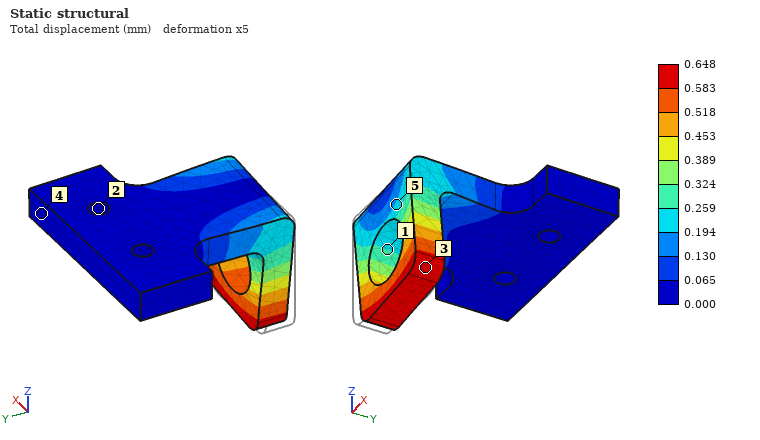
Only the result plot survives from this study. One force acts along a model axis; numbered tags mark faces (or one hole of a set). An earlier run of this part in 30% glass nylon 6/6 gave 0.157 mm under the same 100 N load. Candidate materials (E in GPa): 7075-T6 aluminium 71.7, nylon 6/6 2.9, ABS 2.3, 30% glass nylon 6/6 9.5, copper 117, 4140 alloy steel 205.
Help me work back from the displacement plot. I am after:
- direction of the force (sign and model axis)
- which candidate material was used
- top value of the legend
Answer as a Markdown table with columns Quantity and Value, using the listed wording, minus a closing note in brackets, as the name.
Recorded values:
| Quantity | Value |
|---|---|
| direction of the force | +X |
| which candidate material was used | ABS |
| top value of the legend | 0.648 mm |
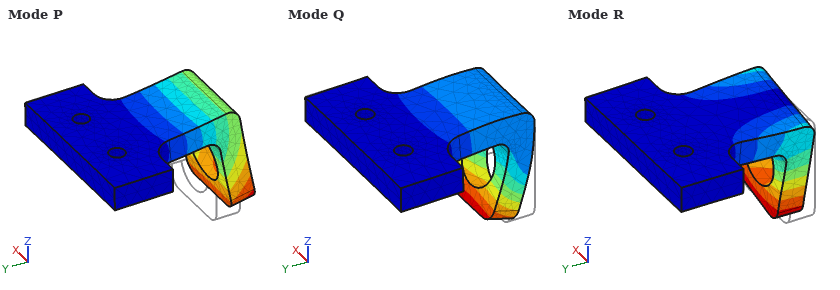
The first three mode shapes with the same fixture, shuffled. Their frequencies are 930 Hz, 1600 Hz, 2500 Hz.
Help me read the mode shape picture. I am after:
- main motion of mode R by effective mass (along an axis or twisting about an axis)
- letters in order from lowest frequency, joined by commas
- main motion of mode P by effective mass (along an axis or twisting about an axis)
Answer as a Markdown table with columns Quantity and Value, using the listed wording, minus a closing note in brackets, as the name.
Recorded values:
| Quantity | Value |
|---|---|
| main motion of mode R by effective mass | along X |
| letters in order from lowest frequency, joined by commas | P, R, Q |
| main motion of mode P by effective mass | along Z |
